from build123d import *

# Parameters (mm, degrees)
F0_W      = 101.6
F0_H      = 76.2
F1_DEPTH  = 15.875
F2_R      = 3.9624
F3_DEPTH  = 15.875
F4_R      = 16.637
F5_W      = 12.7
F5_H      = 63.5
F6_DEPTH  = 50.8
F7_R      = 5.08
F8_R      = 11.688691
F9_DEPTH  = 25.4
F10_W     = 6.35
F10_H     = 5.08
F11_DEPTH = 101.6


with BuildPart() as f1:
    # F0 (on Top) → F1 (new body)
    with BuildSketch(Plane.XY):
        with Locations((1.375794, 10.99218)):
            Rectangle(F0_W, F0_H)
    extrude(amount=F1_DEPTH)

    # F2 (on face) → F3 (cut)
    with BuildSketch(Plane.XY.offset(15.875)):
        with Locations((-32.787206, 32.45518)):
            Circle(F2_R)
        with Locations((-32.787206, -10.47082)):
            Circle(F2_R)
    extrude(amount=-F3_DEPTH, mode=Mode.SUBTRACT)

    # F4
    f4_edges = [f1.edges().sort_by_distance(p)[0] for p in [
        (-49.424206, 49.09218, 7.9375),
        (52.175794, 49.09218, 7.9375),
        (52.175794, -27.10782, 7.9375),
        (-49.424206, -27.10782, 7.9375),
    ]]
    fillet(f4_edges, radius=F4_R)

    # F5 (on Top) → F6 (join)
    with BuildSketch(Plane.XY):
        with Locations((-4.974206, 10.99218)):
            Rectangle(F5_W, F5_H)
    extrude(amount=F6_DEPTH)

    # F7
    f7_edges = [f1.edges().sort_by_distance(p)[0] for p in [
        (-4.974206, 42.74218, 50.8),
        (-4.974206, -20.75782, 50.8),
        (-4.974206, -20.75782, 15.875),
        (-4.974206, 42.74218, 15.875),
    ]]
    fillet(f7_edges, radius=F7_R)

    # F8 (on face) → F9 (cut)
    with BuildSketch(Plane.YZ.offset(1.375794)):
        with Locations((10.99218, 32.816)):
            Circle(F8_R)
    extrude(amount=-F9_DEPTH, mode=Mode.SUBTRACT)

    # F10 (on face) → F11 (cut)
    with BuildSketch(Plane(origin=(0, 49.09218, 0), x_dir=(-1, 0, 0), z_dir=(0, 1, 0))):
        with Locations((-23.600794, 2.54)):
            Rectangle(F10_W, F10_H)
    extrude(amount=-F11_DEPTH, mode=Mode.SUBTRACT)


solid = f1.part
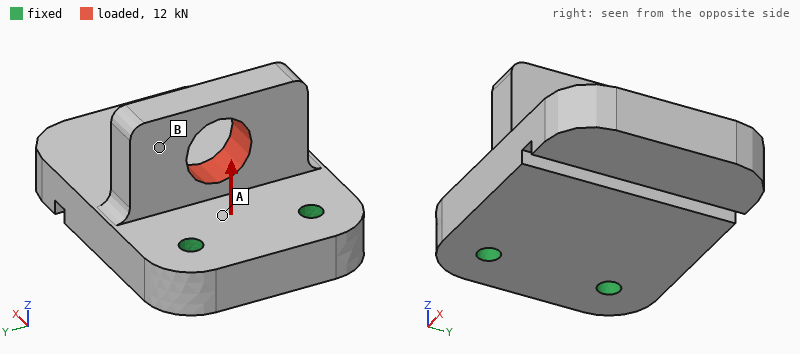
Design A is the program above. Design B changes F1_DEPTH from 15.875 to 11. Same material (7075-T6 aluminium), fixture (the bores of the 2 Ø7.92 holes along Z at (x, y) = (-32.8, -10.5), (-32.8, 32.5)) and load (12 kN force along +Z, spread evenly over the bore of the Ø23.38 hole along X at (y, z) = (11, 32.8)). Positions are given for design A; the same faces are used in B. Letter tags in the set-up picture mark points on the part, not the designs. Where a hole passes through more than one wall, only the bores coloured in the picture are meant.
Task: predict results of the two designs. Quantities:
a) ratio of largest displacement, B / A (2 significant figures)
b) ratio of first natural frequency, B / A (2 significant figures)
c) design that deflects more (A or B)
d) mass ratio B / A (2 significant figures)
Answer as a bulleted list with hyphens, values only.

- 2.6
- 0.70
- B
- 0.77
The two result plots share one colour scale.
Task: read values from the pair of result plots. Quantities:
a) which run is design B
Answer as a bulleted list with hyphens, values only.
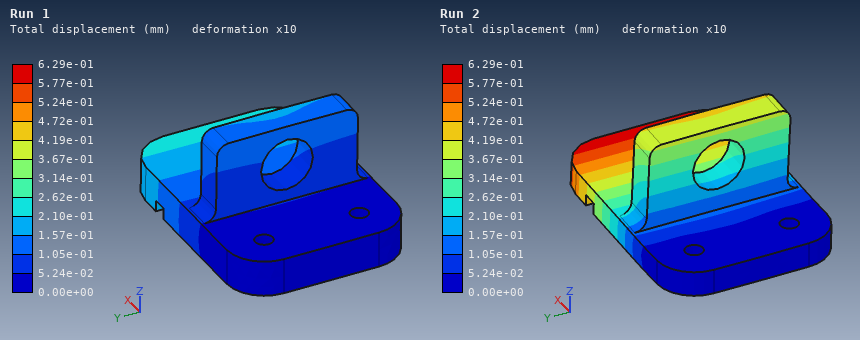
- Run 2
